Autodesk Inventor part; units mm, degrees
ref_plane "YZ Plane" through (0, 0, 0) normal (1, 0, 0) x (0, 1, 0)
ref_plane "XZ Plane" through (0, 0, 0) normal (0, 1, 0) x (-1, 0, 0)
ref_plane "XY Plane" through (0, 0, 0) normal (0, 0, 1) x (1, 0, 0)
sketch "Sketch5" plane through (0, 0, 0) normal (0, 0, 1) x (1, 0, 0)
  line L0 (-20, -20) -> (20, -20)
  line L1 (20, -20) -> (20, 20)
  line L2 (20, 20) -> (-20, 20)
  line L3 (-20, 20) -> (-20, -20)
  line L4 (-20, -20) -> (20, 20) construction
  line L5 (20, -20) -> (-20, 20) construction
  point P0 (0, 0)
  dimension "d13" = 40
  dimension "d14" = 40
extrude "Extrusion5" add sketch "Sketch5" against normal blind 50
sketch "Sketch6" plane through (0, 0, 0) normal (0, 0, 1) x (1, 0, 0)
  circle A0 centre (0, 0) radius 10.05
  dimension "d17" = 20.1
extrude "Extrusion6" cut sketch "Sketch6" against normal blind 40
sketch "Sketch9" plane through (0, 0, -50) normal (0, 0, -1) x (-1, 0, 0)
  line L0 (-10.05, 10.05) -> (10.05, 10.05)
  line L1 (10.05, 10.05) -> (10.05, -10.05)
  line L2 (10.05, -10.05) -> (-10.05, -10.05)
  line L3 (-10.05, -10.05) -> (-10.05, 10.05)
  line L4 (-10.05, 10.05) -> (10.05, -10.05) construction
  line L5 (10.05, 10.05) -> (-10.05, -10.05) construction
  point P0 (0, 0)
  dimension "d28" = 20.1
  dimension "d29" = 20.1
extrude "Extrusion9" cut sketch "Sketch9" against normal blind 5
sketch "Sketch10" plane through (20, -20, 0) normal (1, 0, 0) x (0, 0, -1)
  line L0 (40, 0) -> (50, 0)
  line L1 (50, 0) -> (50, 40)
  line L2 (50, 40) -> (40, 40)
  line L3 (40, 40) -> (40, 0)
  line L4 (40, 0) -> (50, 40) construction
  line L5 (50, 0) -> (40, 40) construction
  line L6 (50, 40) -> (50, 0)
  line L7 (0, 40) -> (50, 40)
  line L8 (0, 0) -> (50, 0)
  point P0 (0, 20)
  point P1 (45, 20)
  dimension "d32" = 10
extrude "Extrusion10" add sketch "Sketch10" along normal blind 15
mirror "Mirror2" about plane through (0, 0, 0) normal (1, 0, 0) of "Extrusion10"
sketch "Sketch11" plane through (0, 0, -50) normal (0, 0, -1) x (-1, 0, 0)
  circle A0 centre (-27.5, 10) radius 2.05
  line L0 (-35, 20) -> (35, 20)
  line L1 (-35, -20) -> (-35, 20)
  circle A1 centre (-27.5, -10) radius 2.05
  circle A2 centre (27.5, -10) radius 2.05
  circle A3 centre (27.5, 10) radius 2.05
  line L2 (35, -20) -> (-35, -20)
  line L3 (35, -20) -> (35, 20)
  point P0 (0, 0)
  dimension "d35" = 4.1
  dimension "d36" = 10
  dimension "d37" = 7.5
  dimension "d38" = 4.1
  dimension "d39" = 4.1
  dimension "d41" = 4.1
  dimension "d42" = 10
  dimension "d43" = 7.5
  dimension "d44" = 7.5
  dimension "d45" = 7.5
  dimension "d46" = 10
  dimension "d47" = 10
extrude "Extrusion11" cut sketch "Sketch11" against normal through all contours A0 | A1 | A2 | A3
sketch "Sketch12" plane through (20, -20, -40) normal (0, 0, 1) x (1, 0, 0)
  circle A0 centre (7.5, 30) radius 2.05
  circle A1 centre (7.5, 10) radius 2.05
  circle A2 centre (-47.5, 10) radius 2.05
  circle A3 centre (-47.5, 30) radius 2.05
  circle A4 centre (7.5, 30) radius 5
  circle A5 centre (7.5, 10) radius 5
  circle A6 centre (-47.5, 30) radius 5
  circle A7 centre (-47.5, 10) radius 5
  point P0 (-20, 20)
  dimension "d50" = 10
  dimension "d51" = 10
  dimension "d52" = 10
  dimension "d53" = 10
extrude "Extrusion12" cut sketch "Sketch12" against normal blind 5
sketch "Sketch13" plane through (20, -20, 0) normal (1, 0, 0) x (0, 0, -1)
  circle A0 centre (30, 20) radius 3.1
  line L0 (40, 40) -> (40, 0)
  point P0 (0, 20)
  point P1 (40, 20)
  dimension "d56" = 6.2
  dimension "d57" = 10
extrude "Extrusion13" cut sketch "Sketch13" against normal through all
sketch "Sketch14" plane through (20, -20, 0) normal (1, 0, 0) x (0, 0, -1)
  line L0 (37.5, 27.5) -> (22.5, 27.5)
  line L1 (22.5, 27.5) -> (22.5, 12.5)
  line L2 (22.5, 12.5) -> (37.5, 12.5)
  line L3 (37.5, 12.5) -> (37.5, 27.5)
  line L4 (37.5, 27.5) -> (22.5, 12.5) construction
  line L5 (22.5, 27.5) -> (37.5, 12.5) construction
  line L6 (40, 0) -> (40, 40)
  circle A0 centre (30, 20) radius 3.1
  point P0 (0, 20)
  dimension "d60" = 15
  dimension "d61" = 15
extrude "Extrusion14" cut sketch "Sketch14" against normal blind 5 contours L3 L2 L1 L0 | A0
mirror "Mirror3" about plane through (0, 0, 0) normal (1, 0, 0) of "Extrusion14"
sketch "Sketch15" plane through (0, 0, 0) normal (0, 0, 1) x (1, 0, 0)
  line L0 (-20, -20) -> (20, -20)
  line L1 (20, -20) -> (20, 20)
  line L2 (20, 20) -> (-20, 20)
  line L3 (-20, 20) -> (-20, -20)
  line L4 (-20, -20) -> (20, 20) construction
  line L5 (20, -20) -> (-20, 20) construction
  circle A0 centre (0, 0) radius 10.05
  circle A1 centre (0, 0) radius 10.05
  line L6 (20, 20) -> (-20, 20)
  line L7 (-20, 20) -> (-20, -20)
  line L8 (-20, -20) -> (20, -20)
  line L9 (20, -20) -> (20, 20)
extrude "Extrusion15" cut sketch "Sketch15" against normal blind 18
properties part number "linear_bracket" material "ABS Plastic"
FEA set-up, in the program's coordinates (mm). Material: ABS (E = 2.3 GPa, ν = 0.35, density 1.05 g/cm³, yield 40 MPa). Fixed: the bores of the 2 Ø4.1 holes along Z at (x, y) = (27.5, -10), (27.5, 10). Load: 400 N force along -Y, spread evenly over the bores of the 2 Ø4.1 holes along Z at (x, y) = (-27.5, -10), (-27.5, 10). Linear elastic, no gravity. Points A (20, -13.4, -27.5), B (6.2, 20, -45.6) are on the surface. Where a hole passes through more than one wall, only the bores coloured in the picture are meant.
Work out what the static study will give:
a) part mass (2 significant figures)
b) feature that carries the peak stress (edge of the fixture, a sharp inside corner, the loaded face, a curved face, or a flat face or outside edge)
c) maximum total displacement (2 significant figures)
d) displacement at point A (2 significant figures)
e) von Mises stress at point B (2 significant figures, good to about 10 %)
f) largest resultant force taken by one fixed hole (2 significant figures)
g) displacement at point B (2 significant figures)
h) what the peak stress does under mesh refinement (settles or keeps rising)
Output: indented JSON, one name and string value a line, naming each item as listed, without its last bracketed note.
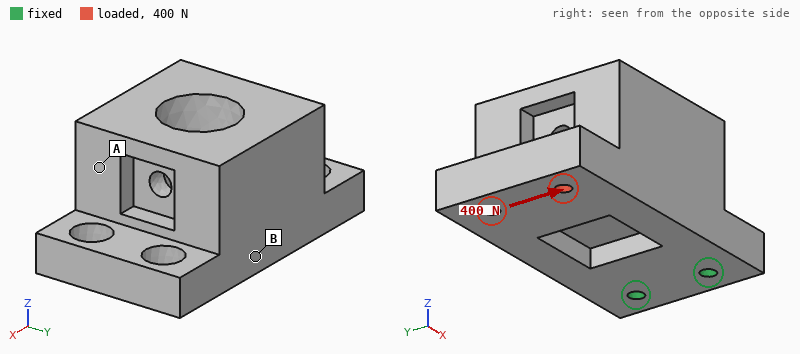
{
  "part mass": "52 g",
  "feature that carries the peak stress": "edge of the fixture",
  "maximum total displacement": "0.67 mm",
  "displacement at point A": "0.14 mm",
  "von Mises stress at point B": "4.8 MPa",
  "largest resultant force taken by one fixed hole": "990 N",
  "displacement at point B": "0.26 mm",
  "what the peak stress does under mesh refinement": "keeps rising"
}
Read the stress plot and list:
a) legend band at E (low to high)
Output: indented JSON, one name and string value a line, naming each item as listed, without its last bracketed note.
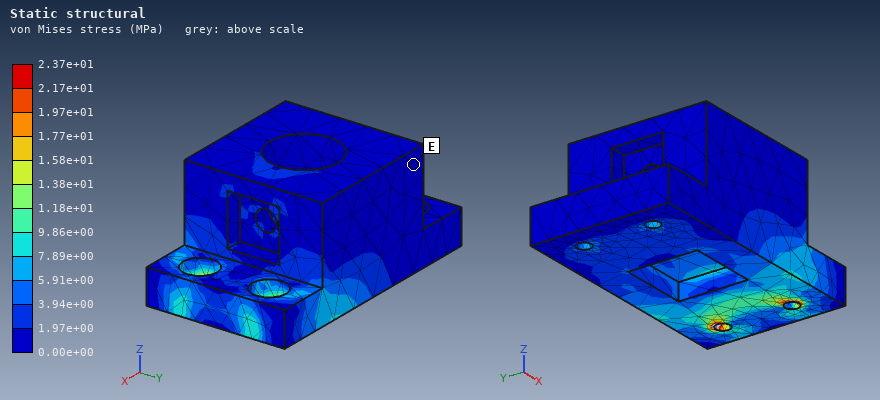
{
  "legend band at E": "0.00e+00 to 1.97e+00 MPa"
}
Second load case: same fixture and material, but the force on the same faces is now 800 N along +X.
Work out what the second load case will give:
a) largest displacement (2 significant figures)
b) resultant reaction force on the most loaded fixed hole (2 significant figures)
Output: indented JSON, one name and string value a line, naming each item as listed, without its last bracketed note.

{
  "largest displacement": "0.34 mm",
  "resultant reaction force on the most loaded fixed hole": "400 N"
}
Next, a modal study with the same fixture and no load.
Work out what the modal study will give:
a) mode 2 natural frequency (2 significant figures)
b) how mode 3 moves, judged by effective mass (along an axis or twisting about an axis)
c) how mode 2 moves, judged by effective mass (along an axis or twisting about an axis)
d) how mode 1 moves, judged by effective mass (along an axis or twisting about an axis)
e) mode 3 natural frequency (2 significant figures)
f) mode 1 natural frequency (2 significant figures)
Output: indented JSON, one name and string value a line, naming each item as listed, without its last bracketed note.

{
  "mode 2 natural frequency": "1100 Hz",
  "how mode 3 moves, judged by effective mass": "twisting about X",
  "how mode 2 moves, judged by effective mass": "along Y",
  "how mode 1 moves, judged by effective mass": "along Z",
  "mode 3 natural frequency": "1300 Hz",
  "mode 1 natural frequency": "320 Hz"
}
